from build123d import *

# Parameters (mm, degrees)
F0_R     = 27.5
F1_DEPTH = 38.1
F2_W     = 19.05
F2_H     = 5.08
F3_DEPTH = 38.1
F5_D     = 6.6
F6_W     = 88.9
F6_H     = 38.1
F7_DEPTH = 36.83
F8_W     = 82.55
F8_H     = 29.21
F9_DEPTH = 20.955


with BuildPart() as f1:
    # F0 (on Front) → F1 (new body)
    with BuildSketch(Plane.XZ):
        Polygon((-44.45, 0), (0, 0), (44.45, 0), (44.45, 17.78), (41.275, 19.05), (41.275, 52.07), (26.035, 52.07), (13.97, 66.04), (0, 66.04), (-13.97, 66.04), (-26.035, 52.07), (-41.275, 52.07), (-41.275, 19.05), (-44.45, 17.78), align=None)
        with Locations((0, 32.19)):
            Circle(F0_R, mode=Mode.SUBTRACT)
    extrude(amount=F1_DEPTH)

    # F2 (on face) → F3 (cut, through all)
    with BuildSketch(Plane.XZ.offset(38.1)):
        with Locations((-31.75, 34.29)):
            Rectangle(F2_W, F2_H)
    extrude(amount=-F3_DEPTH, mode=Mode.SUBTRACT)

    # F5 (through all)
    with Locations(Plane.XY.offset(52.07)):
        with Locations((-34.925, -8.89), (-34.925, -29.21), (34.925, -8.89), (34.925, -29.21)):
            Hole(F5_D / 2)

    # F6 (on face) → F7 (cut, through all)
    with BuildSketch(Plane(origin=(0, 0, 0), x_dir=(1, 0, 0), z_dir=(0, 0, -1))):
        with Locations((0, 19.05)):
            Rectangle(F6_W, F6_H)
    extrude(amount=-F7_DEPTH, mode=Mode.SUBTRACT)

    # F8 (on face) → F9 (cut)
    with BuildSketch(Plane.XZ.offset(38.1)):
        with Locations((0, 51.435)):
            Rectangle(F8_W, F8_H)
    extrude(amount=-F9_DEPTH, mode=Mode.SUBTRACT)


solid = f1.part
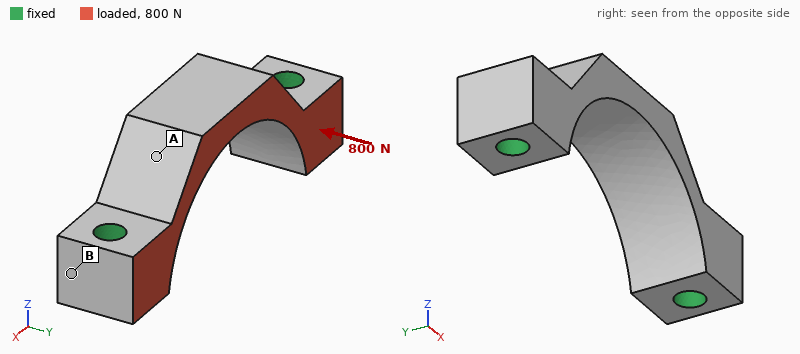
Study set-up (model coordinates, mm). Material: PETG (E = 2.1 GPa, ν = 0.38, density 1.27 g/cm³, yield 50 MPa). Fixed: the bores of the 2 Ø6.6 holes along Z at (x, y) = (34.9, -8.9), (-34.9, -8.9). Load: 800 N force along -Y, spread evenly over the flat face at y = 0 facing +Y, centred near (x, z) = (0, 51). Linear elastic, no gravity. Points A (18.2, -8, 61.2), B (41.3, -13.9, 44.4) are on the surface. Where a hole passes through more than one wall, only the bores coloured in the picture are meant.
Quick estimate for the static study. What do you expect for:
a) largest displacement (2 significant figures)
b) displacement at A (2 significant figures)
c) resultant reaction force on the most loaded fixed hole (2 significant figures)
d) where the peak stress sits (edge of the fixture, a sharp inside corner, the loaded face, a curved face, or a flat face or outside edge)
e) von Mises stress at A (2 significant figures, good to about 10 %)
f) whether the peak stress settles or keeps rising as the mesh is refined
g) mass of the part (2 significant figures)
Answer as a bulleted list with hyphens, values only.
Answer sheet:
- 0.30 mm
- 0.19 mm
- 400 N
- edge of the fixture
- 4.9 MPa
- keeps rising
- 18 g
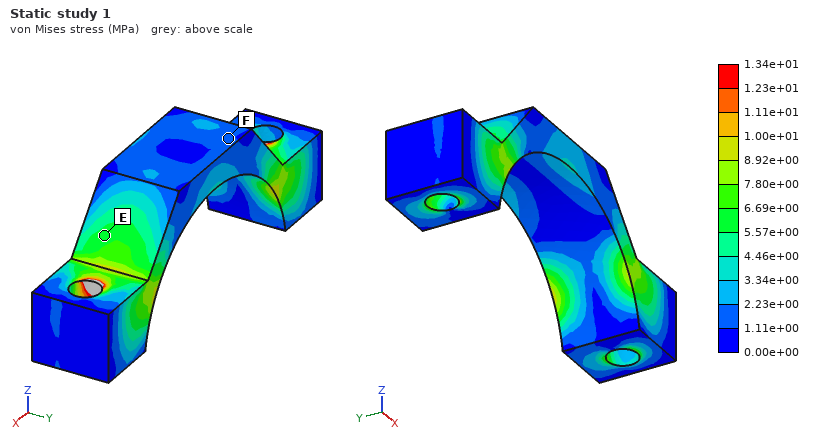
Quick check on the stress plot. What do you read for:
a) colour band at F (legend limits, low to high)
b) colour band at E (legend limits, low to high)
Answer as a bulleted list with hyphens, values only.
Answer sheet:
- 1.11e+00 to 2.23e+00 MPa
- 5.57e+00 to 6.69e+00 MPa
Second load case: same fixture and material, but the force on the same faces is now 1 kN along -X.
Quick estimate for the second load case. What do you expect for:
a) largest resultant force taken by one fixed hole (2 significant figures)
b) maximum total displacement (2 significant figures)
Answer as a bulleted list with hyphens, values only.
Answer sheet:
- 510 N
- 0.14 mm
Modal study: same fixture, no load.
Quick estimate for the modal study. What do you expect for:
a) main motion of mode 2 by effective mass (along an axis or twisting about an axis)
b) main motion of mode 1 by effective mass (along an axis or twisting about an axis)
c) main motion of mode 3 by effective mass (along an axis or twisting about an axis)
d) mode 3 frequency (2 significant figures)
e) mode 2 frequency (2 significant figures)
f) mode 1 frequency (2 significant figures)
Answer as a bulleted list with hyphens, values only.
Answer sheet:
- along X
- along Y
- along Z
- 4700 Hz
- 4000 Hz
- 2200 Hz
